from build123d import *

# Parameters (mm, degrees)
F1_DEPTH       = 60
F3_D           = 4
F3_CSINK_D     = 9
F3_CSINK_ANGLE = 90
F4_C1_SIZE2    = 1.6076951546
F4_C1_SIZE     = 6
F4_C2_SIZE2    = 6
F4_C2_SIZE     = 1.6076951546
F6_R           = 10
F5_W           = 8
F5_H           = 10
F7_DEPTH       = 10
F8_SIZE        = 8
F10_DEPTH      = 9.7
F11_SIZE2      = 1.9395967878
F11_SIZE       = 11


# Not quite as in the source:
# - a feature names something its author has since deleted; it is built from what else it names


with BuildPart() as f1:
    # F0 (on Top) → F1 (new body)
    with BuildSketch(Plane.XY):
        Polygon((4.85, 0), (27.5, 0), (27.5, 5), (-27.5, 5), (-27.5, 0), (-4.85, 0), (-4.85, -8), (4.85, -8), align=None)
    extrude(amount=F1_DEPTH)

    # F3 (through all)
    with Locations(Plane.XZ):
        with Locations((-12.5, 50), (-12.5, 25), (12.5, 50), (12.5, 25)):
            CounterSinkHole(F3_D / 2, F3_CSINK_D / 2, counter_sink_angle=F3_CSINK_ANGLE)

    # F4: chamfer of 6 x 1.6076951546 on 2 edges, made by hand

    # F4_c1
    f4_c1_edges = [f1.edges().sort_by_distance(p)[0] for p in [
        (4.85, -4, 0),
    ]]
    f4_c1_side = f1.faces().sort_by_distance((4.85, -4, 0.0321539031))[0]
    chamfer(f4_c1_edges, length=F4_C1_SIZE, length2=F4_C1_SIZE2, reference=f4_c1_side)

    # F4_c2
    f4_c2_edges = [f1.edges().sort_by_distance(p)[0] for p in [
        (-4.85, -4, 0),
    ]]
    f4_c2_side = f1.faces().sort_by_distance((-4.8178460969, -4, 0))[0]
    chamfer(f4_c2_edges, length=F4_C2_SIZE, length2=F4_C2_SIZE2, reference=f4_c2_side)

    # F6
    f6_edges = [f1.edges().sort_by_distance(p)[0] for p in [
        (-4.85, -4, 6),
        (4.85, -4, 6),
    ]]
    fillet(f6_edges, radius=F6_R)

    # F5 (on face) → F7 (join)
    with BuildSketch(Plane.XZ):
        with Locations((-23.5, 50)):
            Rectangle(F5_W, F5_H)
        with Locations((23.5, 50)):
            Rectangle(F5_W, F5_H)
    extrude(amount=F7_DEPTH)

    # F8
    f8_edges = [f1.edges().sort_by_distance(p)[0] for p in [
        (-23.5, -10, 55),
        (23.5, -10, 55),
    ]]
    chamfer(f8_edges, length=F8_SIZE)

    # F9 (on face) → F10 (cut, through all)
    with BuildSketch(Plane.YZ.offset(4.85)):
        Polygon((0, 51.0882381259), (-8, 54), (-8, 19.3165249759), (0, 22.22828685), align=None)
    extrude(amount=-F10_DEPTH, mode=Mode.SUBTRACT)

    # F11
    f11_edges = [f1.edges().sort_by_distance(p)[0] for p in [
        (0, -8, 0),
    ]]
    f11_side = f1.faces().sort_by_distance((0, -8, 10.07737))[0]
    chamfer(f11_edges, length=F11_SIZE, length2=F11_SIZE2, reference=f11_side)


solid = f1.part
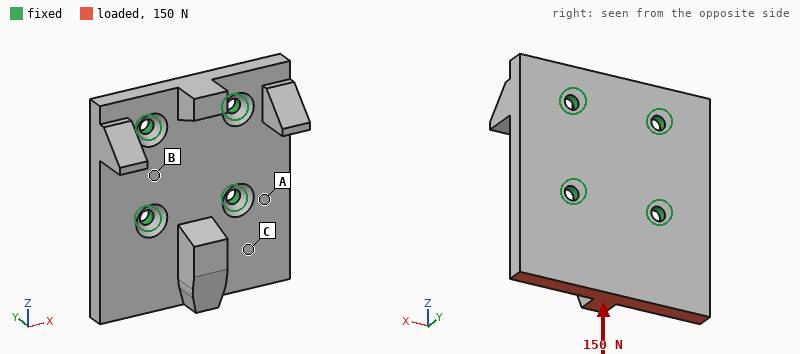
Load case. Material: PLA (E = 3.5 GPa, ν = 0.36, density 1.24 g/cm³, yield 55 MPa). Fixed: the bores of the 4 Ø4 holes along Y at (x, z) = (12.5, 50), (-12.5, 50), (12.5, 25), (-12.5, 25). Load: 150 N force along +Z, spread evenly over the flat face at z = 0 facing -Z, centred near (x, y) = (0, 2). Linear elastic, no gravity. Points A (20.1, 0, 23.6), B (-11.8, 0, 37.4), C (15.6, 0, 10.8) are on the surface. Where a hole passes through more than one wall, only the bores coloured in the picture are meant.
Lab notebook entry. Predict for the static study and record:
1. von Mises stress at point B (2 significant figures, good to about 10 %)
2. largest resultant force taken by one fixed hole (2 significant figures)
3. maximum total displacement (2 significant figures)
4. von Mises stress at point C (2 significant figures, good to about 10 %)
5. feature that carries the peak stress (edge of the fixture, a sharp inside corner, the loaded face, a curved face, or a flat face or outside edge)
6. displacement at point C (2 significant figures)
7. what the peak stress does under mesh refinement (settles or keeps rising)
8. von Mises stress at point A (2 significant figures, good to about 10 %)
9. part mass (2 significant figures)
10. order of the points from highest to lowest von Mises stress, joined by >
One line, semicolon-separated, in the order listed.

0.26 MPa; 52 N; 27 µm; 0.59 MPa; edge of the fixture; 13 µm; keeps rising; 0.88 MPa; 24 g; A > C > B
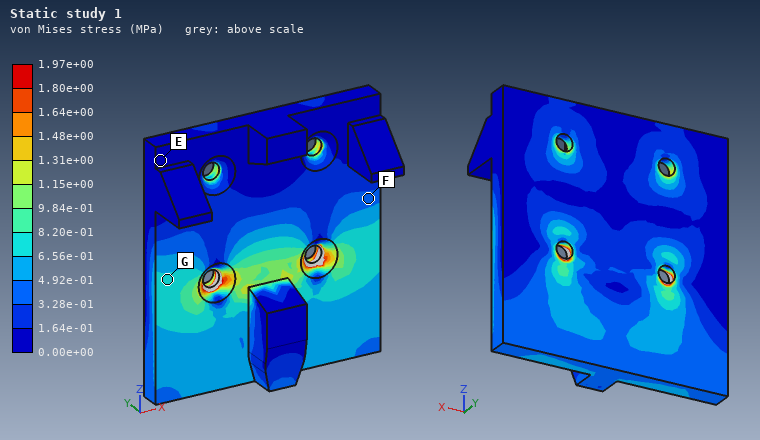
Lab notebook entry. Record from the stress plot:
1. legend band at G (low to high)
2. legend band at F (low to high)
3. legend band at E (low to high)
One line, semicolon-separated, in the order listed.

6.56e-01 to 8.20e-01 MPa; 3.28e-01 to 4.92e-01 MPa; 0.00e+00 to 1.64e-01 MPa
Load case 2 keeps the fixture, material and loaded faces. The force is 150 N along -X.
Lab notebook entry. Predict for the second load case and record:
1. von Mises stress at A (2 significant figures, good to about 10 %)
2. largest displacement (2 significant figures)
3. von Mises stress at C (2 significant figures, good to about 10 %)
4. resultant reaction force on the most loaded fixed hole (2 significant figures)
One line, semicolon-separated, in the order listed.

0.92 MPa; 30 µm; 0.85 MPa; 120 N
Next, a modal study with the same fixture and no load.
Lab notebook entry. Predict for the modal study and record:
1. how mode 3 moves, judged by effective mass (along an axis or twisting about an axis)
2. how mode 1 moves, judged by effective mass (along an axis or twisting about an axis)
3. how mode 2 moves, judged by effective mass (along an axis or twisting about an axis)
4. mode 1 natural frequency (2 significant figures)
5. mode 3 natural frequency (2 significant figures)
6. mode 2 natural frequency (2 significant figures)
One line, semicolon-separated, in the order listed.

along Y; along Y; twisting about Z; 1500 Hz; 3100 Hz; 2500 Hz
